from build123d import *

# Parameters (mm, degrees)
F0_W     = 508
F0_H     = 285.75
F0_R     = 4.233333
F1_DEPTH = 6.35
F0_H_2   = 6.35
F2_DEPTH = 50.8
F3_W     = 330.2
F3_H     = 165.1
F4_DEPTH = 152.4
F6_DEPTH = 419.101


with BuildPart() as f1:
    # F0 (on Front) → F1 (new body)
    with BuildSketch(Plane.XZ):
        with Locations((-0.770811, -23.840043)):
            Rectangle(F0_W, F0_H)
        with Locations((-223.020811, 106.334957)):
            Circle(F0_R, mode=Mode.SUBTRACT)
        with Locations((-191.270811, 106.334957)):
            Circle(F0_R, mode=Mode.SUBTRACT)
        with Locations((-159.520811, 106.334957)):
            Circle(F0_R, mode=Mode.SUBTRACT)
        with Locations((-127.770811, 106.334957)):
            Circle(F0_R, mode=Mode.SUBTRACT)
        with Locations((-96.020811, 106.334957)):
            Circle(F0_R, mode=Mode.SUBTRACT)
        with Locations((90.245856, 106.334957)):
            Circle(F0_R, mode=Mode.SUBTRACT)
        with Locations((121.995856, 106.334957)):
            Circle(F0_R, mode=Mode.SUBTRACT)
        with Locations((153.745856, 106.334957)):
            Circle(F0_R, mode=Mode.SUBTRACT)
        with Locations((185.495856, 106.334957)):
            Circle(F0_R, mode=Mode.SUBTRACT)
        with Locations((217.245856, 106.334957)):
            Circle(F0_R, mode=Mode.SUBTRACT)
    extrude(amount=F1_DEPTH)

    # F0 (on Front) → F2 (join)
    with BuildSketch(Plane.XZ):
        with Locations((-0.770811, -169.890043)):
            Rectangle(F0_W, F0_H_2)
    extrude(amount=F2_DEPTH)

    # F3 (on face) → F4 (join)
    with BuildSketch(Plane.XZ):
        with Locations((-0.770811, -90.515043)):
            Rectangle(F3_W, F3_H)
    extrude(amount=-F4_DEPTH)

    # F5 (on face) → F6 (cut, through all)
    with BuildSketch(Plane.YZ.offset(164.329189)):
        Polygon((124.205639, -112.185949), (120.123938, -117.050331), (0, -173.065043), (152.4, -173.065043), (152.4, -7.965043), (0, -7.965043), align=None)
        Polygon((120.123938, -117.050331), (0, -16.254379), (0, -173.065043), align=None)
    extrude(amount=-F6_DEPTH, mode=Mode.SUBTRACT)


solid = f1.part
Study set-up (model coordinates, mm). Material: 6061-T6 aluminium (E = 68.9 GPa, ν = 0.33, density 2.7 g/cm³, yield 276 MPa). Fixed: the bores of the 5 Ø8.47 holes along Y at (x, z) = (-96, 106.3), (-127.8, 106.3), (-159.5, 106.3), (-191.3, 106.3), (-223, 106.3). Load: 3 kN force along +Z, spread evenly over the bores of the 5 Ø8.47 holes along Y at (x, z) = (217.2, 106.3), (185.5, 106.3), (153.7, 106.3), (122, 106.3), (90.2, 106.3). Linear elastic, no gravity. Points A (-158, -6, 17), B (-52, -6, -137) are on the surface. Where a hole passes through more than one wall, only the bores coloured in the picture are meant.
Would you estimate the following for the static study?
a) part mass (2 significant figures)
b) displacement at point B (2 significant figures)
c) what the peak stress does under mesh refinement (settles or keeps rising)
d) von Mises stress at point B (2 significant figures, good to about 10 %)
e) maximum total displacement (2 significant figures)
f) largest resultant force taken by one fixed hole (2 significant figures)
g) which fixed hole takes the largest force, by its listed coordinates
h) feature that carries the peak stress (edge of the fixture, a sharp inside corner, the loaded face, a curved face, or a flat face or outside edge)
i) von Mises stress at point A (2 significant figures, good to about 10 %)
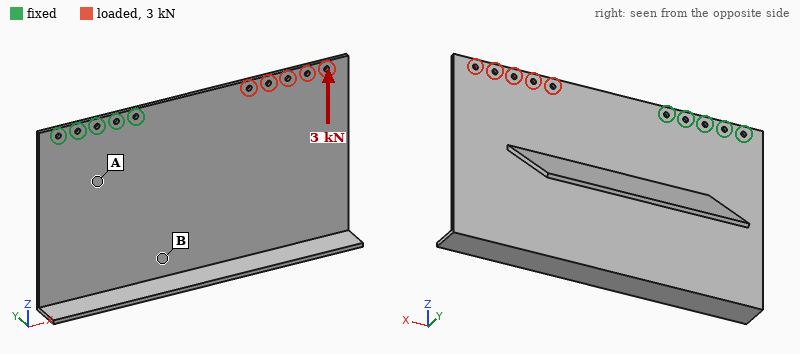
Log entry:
3.8 kg
0.13 mm
keeps rising
3.3 MPa
0.29 mm
7.8 kN
(-96, 106.3)
edge of the fixture
9.0 MPa
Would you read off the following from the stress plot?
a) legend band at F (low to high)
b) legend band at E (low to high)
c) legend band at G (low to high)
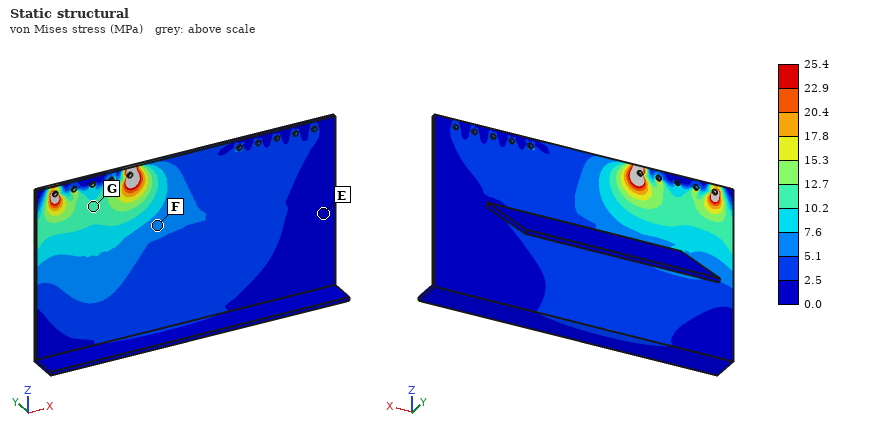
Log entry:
5.1 to 7.6 MPa
0.0 to 2.5 MPa
10.2 to 12.7 MPa
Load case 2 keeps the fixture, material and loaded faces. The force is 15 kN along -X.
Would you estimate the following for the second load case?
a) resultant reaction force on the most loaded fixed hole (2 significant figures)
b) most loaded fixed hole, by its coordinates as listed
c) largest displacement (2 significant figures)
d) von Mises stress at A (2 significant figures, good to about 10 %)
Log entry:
9.1 kN
(-96, 106.3)
0.23 mm
6.1 MPa
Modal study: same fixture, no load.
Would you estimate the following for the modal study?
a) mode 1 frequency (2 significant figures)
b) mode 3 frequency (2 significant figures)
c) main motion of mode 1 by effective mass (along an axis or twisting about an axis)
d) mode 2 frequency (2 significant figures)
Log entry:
26 Hz
120 Hz
along Y
59 Hz
